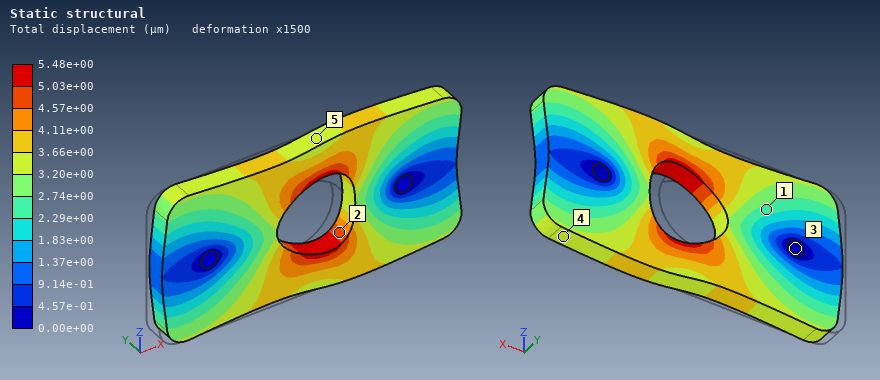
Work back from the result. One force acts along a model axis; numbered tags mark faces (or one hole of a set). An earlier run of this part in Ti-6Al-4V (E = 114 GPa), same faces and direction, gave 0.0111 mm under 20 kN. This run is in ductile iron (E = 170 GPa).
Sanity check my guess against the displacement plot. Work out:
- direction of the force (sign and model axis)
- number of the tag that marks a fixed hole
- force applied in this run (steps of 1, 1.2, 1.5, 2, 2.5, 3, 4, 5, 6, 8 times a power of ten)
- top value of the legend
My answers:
+X
3
15 kN
5.48e+00 µm
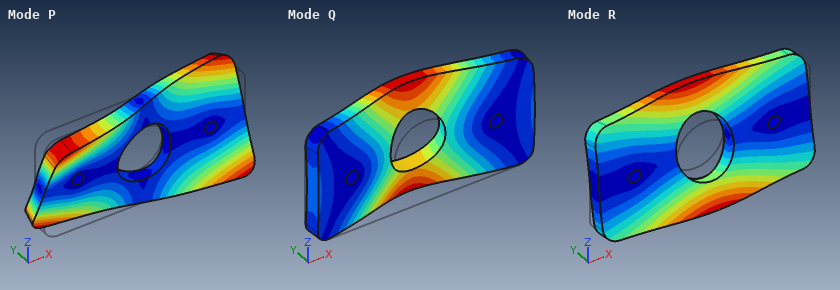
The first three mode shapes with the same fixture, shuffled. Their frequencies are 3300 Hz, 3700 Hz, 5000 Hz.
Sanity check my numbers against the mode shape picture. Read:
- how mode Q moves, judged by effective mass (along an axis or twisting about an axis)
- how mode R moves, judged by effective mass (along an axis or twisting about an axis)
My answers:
along Y
twisting about X
